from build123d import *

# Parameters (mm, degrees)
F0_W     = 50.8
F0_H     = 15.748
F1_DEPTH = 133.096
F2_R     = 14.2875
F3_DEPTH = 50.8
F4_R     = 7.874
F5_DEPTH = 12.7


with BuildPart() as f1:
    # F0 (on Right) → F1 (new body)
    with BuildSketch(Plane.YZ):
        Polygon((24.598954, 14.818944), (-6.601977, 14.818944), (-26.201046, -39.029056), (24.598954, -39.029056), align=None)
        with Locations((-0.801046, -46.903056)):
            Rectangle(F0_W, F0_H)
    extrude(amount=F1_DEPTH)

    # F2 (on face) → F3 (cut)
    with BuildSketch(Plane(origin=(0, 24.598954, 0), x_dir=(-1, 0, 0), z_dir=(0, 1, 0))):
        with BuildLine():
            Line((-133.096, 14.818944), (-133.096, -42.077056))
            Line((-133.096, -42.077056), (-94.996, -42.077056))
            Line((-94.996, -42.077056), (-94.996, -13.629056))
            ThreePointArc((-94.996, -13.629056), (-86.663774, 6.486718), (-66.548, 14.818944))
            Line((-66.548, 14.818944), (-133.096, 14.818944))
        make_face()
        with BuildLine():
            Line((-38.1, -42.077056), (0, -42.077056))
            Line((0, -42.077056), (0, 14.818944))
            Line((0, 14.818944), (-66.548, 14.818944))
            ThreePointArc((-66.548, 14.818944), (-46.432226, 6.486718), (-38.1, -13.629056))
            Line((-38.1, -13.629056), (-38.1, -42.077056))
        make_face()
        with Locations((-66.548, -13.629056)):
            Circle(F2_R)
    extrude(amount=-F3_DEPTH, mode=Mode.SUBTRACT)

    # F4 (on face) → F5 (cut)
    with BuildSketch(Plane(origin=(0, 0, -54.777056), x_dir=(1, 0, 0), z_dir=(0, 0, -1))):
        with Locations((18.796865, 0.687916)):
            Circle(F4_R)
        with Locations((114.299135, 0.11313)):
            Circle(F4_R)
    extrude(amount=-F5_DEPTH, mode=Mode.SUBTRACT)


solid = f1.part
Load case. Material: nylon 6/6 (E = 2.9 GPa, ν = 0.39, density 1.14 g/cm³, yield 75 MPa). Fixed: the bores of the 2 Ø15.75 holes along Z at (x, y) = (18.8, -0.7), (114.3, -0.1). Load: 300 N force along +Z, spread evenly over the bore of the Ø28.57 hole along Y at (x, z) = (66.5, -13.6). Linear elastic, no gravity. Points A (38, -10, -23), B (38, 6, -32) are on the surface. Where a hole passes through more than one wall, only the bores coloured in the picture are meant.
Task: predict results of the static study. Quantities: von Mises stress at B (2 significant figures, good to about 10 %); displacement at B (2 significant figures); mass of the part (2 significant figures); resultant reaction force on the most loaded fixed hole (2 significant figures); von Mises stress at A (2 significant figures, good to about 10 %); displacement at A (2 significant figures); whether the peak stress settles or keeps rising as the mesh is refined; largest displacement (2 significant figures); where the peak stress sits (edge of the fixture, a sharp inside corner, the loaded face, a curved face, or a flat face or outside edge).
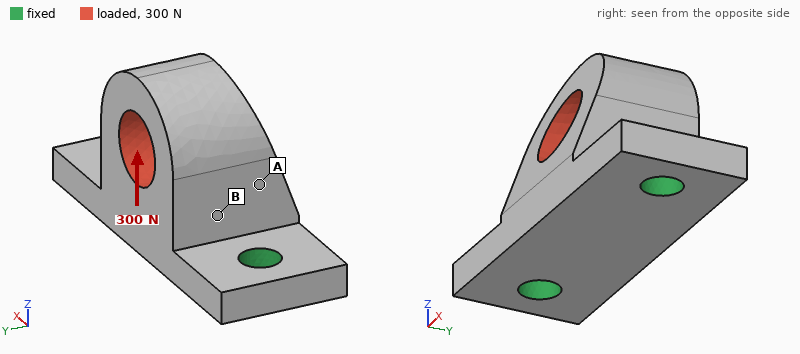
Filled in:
0.37 MPa
14 µm
200 g
160 N
0.18 MPa
12 µm
keeps rising
28 µm
edge of the fixture
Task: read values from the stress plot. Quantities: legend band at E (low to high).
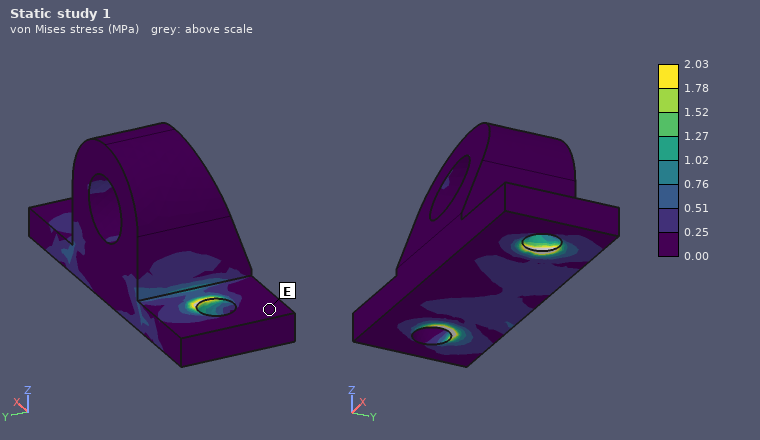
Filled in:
0.00 to 0.25 MPa
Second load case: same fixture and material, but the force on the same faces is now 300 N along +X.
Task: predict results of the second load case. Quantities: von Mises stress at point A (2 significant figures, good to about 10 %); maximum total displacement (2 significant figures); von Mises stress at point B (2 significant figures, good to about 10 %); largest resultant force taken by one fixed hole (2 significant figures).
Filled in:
0.39 MPa
32 µm
0.49 MPa
210 N
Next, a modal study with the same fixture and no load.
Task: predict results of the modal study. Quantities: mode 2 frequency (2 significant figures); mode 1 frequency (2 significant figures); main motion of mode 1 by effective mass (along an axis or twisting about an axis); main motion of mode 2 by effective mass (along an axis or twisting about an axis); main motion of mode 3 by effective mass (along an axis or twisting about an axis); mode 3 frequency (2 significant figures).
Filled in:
1800 Hz
830 Hz
along Y
along X
along Z
1900 Hz
